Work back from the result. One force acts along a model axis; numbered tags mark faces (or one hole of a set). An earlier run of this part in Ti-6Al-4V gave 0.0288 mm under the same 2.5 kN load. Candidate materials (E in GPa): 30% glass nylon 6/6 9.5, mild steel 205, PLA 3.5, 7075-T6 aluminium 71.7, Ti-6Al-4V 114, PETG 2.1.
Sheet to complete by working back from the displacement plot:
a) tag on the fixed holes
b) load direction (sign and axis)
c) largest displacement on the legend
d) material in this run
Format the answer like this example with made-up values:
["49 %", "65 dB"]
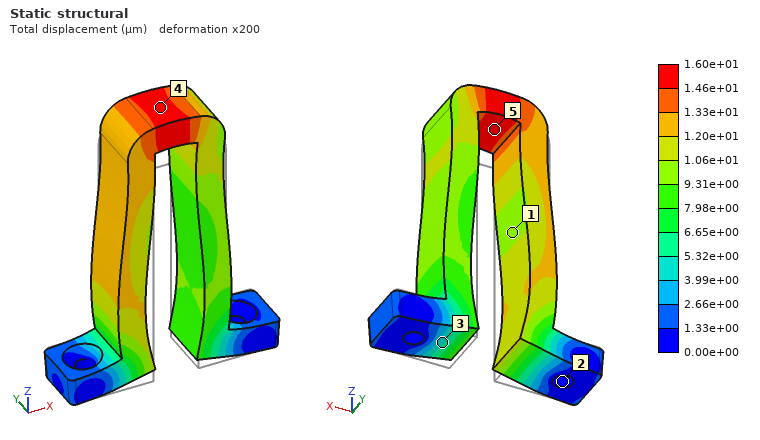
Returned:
["2", "+Z", "1.60e+01 µm", "mild steel"]
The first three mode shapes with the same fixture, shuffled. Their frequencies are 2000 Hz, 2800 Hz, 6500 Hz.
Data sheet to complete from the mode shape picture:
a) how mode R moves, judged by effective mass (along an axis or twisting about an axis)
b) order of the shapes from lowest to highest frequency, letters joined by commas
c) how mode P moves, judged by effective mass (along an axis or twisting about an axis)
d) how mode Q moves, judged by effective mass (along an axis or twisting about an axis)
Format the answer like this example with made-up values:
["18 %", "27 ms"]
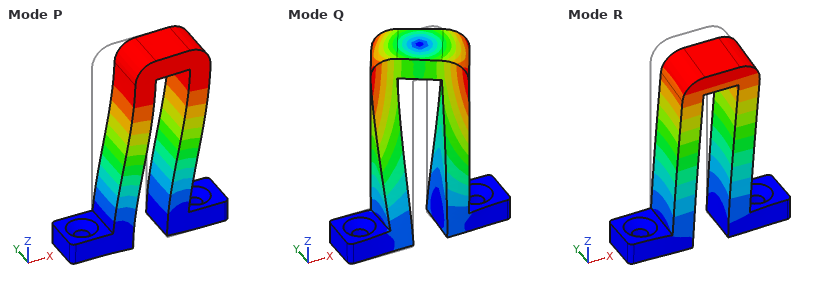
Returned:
["along Y", "R, P, Q", "along X", "twisting about Z"]
